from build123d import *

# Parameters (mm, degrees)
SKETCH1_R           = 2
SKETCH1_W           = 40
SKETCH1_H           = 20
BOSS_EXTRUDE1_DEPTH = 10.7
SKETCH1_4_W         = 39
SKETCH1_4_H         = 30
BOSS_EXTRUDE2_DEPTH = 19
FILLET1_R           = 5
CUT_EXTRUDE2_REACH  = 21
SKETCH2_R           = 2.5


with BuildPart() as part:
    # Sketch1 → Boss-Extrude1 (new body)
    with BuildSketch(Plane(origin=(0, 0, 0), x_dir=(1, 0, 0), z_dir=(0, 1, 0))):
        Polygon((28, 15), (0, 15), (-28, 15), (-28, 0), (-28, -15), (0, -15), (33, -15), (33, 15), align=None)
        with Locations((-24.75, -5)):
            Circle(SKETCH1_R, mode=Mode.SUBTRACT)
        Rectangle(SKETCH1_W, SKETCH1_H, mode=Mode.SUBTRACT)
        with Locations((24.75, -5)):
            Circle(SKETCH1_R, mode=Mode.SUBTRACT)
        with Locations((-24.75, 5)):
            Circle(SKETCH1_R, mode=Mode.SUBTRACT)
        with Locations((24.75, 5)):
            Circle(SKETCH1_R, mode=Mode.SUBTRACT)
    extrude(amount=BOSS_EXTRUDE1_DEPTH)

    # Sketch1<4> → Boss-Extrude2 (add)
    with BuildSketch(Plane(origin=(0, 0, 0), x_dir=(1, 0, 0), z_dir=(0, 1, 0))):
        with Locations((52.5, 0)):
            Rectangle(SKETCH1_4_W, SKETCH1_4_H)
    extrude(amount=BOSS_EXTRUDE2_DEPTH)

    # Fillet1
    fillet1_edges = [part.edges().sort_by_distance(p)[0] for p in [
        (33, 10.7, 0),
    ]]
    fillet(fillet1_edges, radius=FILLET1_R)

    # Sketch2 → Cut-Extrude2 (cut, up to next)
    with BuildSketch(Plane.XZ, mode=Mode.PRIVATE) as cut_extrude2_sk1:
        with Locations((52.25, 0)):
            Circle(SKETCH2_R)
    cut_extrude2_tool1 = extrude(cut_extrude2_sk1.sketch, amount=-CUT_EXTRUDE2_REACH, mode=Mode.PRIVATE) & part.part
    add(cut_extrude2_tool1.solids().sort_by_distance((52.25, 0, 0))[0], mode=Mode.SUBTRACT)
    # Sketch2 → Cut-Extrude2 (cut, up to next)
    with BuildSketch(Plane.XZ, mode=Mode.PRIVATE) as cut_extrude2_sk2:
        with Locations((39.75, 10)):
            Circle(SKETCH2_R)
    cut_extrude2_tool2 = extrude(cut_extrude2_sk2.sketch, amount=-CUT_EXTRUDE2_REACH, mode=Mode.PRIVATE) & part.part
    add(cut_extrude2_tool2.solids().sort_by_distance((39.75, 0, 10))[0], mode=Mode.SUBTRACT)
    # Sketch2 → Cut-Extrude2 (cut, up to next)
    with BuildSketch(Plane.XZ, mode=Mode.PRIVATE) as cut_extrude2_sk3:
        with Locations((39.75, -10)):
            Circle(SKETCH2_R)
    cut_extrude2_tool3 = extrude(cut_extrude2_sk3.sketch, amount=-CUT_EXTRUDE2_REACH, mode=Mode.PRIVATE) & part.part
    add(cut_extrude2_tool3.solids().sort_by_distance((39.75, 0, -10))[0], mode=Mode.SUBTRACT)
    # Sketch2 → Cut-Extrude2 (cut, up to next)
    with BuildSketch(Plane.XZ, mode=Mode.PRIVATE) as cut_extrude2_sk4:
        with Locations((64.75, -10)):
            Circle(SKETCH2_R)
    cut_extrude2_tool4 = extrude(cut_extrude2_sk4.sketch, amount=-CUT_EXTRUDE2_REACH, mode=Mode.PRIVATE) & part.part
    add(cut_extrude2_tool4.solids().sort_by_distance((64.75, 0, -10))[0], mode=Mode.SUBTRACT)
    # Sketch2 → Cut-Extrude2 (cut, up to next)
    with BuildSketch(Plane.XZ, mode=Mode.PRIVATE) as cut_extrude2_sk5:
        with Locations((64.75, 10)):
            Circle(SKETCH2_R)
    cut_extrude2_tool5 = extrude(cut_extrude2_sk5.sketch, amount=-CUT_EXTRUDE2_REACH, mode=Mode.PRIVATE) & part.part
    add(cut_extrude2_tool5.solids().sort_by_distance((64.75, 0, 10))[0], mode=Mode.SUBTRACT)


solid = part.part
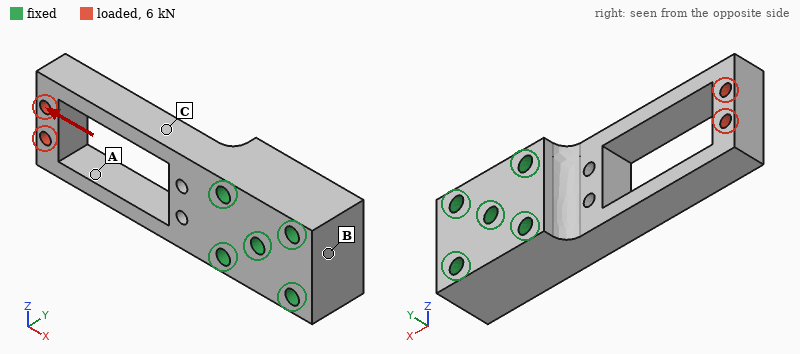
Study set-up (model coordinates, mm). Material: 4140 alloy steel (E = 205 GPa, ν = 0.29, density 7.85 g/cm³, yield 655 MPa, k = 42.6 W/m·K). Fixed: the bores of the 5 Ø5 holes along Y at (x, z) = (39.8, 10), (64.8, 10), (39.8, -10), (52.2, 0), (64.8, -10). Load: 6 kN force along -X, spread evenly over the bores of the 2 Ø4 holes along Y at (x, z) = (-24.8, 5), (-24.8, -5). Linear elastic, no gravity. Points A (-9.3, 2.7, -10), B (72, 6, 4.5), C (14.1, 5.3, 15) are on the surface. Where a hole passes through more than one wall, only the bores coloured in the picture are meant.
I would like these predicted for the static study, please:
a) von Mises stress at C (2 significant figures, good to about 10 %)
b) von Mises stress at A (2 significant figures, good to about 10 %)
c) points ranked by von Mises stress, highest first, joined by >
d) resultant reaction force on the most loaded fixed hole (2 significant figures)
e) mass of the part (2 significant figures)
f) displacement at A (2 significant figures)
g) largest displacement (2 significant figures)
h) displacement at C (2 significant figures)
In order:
67 MPa
110 MPa
A > C > B
2.8 kN
240 g
21 µm
37 µm
9.3 µm
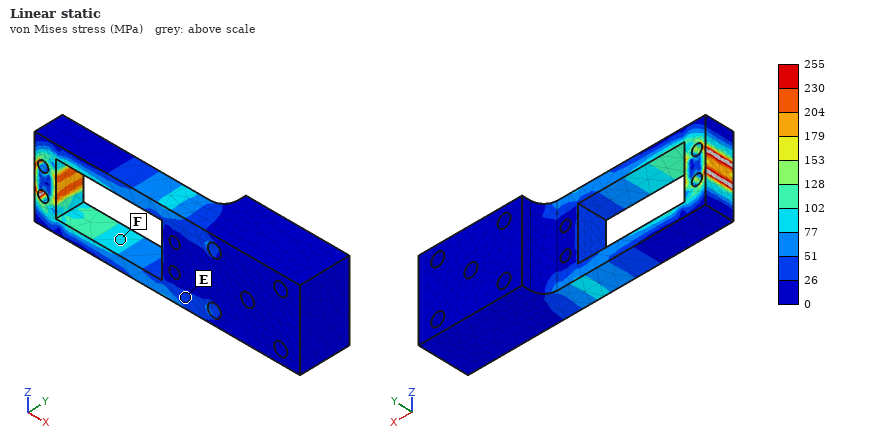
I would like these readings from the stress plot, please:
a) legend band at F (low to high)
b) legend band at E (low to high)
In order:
77 to 102 MPa
26 to 51 MPa
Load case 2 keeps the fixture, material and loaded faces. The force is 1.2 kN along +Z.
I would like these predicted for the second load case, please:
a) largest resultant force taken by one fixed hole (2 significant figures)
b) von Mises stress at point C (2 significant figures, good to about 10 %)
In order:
3.4 kN
220 MPa
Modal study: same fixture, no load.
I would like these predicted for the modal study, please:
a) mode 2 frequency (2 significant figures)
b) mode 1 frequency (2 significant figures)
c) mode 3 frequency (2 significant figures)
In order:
2000 Hz
2000 Hz
4400 Hz
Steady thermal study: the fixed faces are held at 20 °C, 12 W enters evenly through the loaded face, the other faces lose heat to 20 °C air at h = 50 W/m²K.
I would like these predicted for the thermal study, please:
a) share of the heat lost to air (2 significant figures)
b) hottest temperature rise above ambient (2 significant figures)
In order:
66 %
75 K
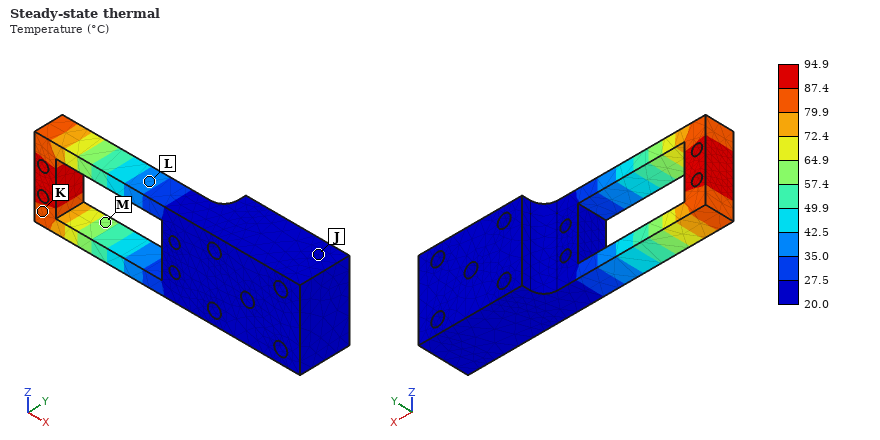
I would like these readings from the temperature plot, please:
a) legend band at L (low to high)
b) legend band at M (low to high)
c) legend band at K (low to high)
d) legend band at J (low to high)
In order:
35.0 to 42.5 °C
57.4 to 64.9 °C
79.9 to 87.4 °C
20.0 to 27.5 °C
